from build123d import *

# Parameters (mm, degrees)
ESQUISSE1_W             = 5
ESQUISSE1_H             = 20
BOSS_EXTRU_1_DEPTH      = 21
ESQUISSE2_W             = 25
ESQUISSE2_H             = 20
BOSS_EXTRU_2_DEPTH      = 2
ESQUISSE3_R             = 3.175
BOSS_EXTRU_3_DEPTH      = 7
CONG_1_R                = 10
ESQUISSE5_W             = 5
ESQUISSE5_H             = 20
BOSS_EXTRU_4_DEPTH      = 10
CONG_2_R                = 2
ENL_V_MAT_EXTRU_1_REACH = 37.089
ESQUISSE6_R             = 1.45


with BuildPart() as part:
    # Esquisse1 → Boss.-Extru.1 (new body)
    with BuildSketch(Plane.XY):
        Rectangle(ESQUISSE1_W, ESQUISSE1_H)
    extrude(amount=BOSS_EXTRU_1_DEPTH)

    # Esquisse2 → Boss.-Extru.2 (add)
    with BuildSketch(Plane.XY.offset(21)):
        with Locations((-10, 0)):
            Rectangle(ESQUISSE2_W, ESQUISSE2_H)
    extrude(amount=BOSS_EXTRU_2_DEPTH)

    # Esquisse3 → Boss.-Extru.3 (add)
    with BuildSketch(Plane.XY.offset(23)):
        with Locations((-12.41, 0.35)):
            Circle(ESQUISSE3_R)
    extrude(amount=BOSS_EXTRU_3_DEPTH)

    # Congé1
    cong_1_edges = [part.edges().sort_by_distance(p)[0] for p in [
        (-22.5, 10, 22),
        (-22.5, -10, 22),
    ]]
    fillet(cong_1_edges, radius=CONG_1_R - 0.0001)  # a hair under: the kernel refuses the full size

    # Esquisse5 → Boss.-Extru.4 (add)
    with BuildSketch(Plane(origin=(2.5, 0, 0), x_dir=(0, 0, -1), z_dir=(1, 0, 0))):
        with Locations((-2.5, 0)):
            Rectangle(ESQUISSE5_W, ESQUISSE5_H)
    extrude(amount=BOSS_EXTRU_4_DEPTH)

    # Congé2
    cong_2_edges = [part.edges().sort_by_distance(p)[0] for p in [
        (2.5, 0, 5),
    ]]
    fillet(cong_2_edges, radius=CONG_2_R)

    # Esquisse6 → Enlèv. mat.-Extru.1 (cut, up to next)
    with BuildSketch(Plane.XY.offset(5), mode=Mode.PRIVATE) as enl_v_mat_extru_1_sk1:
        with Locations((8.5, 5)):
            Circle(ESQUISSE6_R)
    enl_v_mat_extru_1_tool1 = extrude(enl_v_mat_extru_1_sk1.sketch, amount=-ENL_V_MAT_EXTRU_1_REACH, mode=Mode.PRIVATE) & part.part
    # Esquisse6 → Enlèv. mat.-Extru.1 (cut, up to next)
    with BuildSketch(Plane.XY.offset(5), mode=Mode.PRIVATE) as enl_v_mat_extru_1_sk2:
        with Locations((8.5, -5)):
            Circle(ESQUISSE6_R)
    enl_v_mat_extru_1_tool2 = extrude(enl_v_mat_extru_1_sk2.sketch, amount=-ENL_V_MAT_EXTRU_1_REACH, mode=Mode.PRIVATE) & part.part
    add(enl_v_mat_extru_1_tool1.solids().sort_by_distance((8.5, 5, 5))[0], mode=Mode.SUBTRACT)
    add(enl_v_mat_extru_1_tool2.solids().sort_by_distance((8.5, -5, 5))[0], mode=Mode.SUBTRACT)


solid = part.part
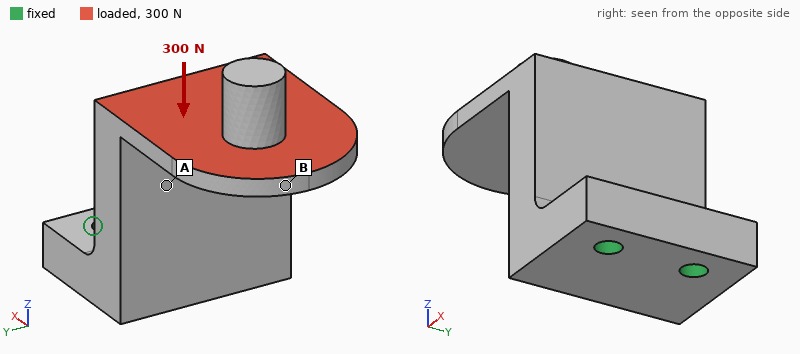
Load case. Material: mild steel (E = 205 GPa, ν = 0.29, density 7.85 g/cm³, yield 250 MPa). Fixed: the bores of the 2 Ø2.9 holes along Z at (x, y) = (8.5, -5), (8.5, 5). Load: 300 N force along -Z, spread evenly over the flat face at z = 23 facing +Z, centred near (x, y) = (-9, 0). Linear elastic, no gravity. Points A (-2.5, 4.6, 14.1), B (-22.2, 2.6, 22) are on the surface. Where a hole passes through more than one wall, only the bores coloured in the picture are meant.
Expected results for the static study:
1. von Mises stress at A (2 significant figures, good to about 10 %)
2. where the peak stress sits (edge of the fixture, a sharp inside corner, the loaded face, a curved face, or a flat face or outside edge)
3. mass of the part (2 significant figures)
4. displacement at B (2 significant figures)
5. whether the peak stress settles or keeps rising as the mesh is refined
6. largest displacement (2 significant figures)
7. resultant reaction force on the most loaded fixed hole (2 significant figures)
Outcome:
33 MPa
edge of the fixture
33 g
0.12 mm
keeps rising
0.13 mm
150 N
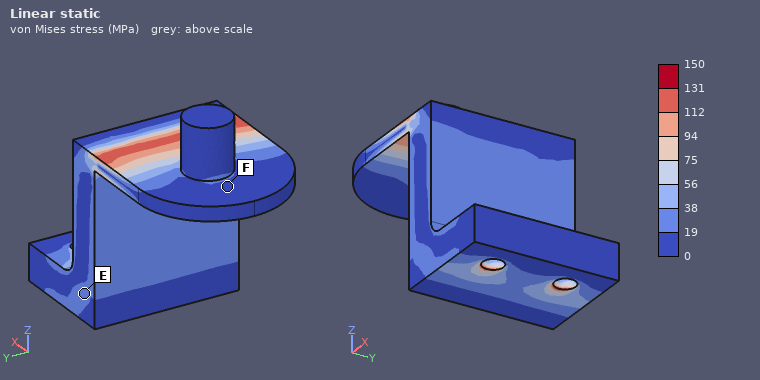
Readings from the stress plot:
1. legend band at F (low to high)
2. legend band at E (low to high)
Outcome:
0 to 19 MPa
19 to 38 MPa
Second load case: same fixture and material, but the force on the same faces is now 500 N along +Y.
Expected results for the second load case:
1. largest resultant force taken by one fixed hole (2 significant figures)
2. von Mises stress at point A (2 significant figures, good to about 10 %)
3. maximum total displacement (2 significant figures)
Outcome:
1.0 kN
51 MPa
37 µm
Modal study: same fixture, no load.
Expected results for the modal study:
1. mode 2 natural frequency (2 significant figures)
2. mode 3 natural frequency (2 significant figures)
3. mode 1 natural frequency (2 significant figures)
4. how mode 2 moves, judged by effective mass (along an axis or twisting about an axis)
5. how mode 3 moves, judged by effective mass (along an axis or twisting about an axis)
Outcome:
5900 Hz
6600 Hz
2800 Hz
along X
along Y
